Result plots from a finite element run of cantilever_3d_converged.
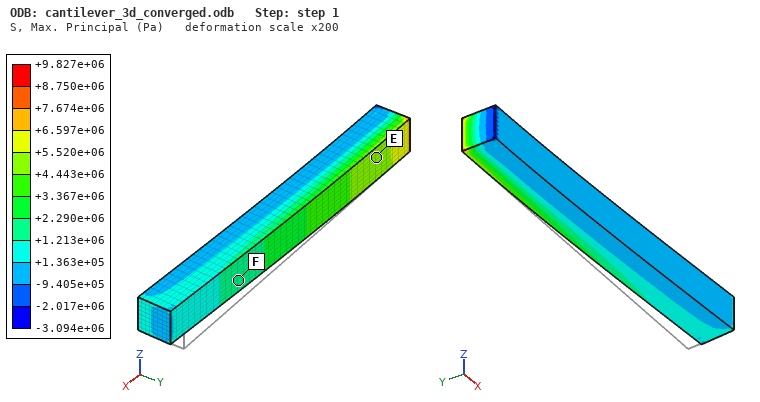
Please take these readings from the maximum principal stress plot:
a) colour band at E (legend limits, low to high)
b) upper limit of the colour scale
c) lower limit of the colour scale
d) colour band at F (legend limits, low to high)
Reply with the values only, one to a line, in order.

+4.443e+06 to +5.520e+06 Pa
+9.827e+06 Pa
-3.094e+06 Pa
+1.213e+06 to +2.290e+06 Pa
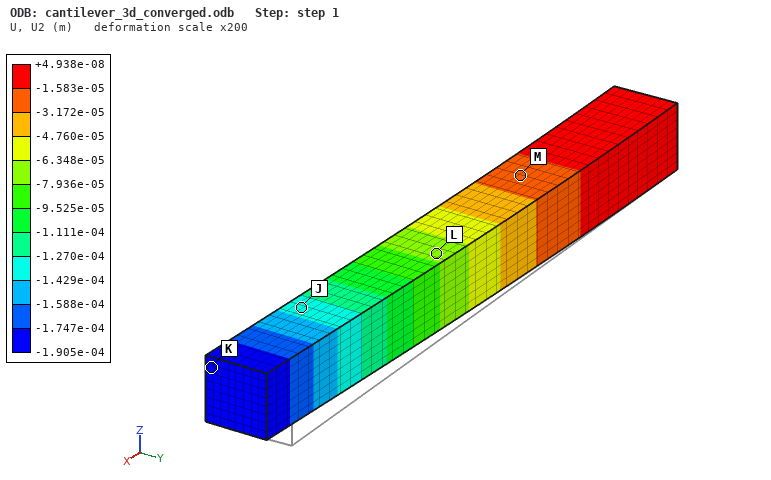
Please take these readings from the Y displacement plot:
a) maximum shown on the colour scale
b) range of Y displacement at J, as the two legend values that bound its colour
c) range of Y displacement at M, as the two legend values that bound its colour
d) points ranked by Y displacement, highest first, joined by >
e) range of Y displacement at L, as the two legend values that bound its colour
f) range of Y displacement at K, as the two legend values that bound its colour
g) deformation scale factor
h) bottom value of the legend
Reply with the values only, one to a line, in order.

+4.938e-08 m
-1.429e-04 to -1.270e-04 m
-3.172e-05 to -1.583e-05 m
M > L > J > K
-7.936e-05 to -6.348e-05 m
-1.905e-04 to -1.747e-04 m
200
-1.905e-04 m
